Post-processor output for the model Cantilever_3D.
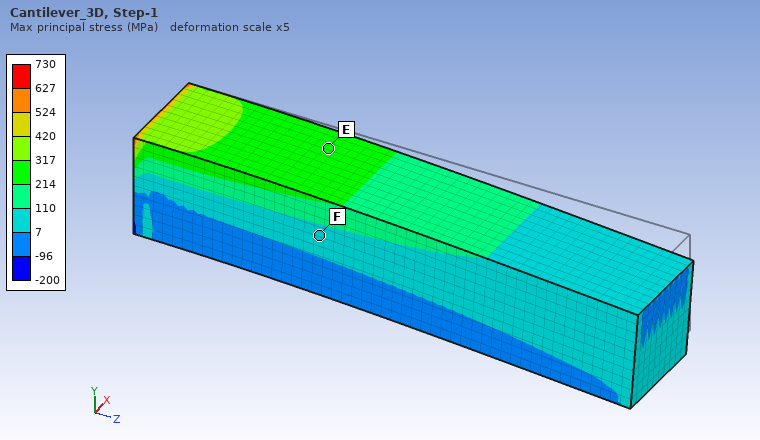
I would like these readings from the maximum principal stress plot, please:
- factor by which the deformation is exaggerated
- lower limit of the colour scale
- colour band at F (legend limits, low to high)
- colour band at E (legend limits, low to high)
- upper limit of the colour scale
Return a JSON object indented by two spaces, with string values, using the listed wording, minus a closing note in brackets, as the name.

{
  "factor by which the deformation is exaggerated": "5",
  "lower limit of the colour scale": "-200 MPa",
  "colour band at F": "7 to 110 MPa",
  "colour band at E": "214 to 317 MPa",
  "upper limit of the colour scale": "730 MPa"
}
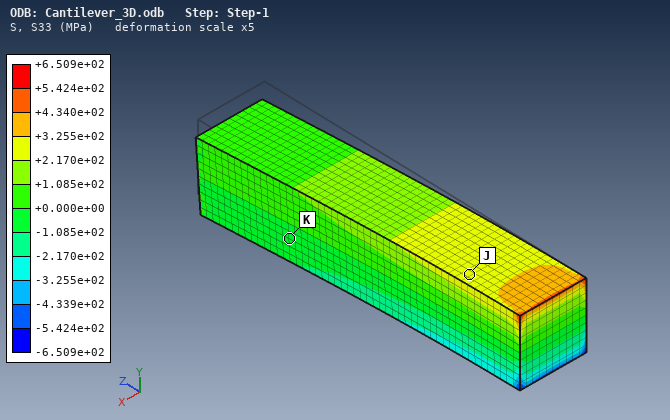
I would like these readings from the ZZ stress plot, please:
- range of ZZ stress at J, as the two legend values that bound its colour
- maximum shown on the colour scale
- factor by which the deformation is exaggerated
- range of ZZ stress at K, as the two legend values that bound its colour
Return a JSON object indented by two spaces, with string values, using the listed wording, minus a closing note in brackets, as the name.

{
  "range of ZZ stress at J, as the two legend values that bound its colour": "+2.170e+02 to +3.255e+02 MPa",
  "maximum shown on the colour scale": "+6.509e+02 MPa",
  "factor by which the deformation is exaggerated": "5",
  "range of ZZ stress at K, as the two legend values that bound its colour": "-1.085e+02 to +0.000e+00 MPa"
}
